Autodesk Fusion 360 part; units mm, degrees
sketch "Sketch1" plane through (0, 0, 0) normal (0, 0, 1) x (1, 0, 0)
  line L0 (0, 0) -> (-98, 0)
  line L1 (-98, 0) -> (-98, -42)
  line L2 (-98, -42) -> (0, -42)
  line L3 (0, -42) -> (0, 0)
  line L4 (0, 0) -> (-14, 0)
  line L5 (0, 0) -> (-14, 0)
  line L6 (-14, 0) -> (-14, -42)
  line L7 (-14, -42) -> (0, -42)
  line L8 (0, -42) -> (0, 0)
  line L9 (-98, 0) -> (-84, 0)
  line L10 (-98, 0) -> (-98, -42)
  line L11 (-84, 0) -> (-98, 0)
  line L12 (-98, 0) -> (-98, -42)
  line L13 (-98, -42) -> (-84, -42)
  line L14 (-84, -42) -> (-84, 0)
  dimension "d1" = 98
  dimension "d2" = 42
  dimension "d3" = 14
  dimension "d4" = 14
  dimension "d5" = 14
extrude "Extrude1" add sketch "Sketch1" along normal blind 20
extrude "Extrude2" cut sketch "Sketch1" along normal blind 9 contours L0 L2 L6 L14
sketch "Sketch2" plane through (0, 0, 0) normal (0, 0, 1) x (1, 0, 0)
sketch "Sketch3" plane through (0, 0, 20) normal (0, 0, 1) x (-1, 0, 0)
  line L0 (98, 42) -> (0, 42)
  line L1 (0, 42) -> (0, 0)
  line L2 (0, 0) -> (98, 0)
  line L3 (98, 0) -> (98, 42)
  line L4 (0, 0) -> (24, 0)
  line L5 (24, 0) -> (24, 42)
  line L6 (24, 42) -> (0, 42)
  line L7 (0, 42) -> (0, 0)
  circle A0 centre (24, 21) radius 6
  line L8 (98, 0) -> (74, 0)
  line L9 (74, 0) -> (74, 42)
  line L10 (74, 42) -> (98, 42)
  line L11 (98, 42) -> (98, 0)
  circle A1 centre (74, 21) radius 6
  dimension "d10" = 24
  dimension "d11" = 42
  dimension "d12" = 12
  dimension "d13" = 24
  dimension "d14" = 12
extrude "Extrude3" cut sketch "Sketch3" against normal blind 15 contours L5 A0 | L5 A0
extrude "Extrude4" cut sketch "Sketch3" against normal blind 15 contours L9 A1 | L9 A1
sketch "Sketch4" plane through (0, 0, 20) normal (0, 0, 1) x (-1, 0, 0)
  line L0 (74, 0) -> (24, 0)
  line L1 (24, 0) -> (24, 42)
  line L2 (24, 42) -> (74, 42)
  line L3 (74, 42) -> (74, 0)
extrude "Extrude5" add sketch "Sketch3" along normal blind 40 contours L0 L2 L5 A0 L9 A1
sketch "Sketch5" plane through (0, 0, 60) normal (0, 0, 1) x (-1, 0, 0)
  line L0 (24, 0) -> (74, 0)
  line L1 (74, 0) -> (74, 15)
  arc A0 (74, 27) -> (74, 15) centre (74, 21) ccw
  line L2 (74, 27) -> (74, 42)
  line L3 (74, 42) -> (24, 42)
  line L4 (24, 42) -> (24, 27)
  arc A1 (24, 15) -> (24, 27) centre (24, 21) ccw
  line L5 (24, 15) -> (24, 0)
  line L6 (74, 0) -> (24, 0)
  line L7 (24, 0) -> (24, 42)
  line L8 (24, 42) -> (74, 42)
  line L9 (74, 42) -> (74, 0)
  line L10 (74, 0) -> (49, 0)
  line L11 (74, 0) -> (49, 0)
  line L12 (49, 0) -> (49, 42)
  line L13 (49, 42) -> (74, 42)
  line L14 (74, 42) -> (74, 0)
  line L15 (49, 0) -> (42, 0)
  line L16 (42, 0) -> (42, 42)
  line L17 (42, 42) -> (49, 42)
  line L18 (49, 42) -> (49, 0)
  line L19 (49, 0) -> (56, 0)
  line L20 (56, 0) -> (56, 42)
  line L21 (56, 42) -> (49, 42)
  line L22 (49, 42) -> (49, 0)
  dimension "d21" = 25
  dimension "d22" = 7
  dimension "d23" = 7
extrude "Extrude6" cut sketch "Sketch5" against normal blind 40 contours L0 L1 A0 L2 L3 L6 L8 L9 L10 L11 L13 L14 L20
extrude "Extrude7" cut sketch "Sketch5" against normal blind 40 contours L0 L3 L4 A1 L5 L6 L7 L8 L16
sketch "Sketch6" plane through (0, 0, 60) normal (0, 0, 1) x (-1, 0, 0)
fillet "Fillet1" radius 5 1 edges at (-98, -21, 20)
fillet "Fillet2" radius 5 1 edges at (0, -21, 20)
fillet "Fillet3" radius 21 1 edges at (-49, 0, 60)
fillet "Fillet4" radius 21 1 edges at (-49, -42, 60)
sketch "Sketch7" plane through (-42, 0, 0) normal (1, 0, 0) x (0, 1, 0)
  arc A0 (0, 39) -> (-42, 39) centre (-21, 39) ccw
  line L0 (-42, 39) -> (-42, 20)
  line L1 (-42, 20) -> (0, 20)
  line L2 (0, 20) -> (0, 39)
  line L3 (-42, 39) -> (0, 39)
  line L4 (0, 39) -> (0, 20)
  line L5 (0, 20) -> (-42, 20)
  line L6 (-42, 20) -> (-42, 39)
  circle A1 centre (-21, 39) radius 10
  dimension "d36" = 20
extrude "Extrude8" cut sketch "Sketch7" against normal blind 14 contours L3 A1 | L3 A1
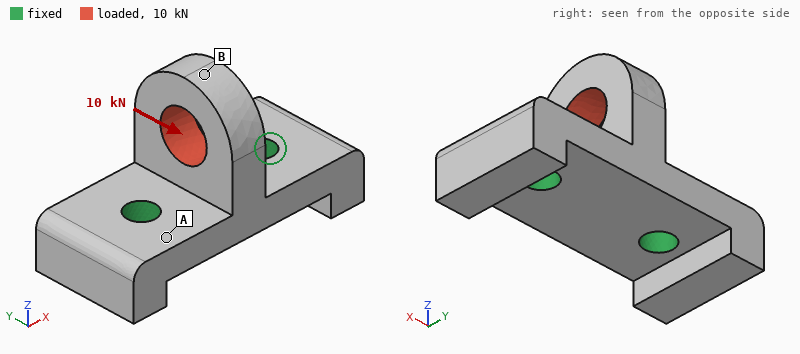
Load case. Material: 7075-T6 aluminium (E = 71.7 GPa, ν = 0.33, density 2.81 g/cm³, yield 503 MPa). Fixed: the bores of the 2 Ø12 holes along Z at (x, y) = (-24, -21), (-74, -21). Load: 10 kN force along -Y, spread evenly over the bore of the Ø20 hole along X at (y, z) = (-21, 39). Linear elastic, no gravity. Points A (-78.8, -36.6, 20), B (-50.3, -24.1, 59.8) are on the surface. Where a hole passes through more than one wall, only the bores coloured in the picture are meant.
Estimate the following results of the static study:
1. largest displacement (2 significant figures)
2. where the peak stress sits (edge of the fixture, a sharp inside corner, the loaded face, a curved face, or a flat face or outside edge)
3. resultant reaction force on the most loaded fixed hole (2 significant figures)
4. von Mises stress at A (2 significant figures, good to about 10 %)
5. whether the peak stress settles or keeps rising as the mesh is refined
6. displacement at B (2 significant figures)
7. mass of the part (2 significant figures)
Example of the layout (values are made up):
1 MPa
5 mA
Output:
0.22 mm
edge of the fixture
5.0 kN
39 MPa
keeps rising
0.22 mm
190 g
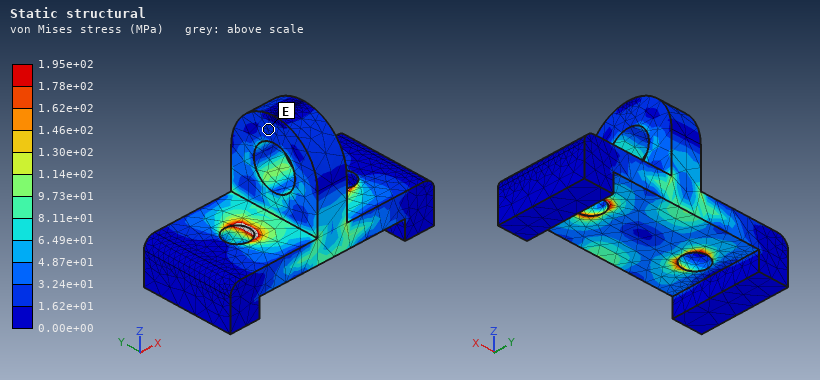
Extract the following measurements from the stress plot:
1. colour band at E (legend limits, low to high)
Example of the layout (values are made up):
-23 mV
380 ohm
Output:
1.62e+01 to 3.24e+01 MPa
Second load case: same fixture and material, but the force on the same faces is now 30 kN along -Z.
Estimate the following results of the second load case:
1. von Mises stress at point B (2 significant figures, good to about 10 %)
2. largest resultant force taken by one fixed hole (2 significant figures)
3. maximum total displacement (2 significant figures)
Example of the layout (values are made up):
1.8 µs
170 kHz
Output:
65 MPa
15 kN
0.11 mm
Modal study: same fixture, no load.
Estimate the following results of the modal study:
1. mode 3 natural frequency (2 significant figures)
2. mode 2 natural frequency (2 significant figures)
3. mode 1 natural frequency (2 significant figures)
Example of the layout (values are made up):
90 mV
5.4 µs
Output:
10 kHz
5600 Hz
5500 Hz
